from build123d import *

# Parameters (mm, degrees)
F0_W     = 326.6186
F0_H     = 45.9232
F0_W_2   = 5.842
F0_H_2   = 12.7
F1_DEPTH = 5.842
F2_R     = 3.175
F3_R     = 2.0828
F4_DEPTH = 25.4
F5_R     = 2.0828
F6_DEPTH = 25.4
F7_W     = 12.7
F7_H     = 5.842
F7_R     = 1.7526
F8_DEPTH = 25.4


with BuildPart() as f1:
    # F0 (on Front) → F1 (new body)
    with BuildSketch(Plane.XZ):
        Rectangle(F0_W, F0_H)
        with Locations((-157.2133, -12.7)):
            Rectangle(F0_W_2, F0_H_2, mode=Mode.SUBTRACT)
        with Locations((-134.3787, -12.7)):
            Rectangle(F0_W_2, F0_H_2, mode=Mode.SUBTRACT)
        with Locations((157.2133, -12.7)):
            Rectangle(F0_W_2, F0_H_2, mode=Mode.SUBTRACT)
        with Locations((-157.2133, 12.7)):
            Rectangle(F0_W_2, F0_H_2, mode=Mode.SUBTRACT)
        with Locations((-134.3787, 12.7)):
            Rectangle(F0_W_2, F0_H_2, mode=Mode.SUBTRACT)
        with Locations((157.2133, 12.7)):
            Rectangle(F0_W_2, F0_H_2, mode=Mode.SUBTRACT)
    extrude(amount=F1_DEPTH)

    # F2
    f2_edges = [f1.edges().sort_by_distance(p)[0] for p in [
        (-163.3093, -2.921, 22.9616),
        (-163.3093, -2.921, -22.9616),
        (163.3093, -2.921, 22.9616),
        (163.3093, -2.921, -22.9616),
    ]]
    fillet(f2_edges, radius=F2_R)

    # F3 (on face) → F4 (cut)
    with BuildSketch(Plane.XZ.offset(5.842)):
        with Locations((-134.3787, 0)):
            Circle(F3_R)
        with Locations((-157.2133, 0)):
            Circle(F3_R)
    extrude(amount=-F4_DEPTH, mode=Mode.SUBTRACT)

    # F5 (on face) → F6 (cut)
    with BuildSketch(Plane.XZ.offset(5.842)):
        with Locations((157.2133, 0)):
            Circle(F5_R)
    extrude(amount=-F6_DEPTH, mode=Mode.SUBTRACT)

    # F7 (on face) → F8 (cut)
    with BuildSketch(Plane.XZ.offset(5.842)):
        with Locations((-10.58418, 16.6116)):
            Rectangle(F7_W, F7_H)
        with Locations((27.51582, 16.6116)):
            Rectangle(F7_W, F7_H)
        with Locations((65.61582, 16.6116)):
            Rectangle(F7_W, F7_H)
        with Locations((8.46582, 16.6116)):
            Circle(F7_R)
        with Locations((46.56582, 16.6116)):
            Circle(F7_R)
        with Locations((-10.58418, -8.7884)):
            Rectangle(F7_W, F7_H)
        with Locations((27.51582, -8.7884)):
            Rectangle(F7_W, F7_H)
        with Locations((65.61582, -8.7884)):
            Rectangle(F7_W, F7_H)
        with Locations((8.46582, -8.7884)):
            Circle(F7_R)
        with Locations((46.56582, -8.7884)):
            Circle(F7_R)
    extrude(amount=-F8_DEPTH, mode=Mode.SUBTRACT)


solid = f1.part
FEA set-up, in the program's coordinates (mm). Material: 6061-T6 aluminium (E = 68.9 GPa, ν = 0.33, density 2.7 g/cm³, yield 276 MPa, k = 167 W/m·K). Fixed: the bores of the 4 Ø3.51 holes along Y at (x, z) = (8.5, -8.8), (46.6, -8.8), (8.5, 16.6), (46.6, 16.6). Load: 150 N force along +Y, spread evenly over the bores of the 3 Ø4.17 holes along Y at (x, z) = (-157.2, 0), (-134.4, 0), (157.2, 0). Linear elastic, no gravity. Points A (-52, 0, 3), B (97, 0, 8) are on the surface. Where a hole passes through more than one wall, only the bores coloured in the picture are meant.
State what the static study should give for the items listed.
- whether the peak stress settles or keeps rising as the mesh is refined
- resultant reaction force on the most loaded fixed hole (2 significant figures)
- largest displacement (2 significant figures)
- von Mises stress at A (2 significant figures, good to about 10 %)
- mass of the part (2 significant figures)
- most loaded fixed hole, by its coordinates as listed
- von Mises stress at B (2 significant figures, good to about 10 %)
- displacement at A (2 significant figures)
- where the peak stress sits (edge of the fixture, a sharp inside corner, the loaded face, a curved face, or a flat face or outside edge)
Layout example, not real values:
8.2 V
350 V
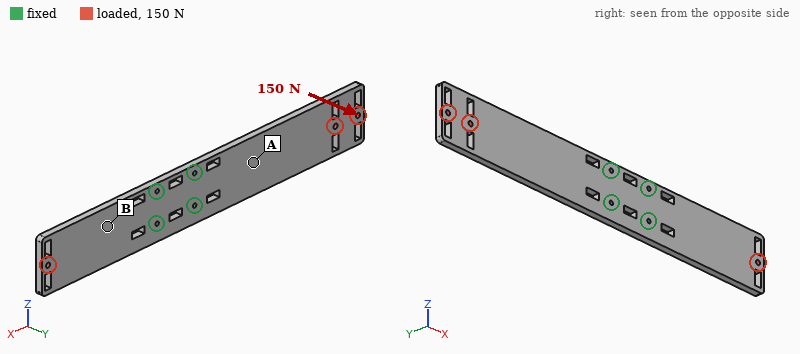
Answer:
keeps rising
130 N
3.0 mm
36 MPa
220 g
(8.5, -8.8)
11 MPa
0.55 mm
edge of the fixture
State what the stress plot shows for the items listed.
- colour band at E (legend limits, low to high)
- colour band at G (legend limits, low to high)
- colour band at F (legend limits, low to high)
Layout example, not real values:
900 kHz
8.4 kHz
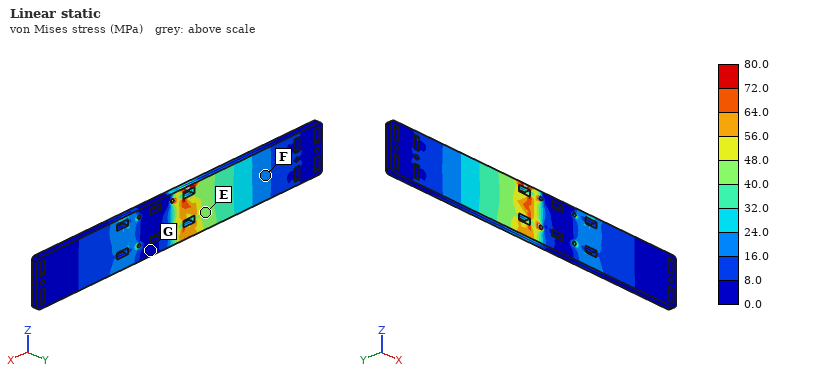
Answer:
40.0 to 48.0 MPa
0.0 to 8.0 MPa
16.0 to 24.0 MPa
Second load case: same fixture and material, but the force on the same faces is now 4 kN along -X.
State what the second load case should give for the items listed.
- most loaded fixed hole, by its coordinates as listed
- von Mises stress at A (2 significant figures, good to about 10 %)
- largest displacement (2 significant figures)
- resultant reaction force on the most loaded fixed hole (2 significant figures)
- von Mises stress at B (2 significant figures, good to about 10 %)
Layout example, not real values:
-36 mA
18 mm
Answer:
(8.5, -8.8)
10.0 MPa
32 µm
1.5 kN
5.0 MPa
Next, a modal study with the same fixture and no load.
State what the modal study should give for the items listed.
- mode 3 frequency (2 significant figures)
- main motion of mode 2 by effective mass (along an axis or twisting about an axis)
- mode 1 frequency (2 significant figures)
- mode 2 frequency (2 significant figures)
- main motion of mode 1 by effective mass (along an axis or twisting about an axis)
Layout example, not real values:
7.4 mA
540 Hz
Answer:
1000 Hz
along Y
160 Hz
340 Hz
along Y
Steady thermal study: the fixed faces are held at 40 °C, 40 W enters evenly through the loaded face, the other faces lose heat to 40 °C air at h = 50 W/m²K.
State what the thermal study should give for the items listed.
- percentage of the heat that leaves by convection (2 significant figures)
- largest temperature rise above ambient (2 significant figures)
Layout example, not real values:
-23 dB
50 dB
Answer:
66 %
52 K
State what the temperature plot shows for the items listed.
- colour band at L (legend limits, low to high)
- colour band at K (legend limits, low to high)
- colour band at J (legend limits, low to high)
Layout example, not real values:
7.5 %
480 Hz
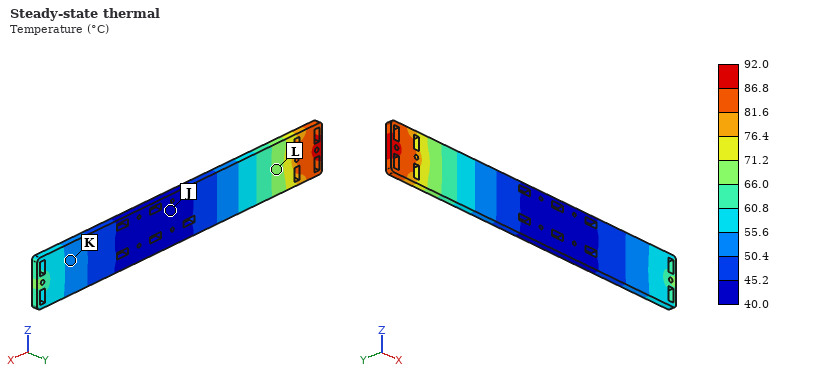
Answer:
66.0 to 71.2 °C
50.4 to 55.6 °C
40.0 to 45.2 °C
